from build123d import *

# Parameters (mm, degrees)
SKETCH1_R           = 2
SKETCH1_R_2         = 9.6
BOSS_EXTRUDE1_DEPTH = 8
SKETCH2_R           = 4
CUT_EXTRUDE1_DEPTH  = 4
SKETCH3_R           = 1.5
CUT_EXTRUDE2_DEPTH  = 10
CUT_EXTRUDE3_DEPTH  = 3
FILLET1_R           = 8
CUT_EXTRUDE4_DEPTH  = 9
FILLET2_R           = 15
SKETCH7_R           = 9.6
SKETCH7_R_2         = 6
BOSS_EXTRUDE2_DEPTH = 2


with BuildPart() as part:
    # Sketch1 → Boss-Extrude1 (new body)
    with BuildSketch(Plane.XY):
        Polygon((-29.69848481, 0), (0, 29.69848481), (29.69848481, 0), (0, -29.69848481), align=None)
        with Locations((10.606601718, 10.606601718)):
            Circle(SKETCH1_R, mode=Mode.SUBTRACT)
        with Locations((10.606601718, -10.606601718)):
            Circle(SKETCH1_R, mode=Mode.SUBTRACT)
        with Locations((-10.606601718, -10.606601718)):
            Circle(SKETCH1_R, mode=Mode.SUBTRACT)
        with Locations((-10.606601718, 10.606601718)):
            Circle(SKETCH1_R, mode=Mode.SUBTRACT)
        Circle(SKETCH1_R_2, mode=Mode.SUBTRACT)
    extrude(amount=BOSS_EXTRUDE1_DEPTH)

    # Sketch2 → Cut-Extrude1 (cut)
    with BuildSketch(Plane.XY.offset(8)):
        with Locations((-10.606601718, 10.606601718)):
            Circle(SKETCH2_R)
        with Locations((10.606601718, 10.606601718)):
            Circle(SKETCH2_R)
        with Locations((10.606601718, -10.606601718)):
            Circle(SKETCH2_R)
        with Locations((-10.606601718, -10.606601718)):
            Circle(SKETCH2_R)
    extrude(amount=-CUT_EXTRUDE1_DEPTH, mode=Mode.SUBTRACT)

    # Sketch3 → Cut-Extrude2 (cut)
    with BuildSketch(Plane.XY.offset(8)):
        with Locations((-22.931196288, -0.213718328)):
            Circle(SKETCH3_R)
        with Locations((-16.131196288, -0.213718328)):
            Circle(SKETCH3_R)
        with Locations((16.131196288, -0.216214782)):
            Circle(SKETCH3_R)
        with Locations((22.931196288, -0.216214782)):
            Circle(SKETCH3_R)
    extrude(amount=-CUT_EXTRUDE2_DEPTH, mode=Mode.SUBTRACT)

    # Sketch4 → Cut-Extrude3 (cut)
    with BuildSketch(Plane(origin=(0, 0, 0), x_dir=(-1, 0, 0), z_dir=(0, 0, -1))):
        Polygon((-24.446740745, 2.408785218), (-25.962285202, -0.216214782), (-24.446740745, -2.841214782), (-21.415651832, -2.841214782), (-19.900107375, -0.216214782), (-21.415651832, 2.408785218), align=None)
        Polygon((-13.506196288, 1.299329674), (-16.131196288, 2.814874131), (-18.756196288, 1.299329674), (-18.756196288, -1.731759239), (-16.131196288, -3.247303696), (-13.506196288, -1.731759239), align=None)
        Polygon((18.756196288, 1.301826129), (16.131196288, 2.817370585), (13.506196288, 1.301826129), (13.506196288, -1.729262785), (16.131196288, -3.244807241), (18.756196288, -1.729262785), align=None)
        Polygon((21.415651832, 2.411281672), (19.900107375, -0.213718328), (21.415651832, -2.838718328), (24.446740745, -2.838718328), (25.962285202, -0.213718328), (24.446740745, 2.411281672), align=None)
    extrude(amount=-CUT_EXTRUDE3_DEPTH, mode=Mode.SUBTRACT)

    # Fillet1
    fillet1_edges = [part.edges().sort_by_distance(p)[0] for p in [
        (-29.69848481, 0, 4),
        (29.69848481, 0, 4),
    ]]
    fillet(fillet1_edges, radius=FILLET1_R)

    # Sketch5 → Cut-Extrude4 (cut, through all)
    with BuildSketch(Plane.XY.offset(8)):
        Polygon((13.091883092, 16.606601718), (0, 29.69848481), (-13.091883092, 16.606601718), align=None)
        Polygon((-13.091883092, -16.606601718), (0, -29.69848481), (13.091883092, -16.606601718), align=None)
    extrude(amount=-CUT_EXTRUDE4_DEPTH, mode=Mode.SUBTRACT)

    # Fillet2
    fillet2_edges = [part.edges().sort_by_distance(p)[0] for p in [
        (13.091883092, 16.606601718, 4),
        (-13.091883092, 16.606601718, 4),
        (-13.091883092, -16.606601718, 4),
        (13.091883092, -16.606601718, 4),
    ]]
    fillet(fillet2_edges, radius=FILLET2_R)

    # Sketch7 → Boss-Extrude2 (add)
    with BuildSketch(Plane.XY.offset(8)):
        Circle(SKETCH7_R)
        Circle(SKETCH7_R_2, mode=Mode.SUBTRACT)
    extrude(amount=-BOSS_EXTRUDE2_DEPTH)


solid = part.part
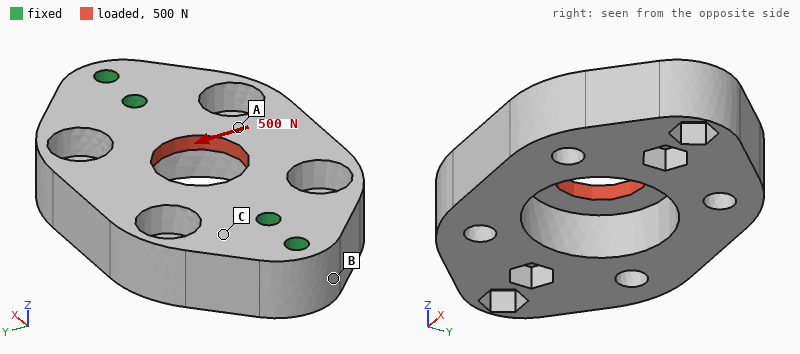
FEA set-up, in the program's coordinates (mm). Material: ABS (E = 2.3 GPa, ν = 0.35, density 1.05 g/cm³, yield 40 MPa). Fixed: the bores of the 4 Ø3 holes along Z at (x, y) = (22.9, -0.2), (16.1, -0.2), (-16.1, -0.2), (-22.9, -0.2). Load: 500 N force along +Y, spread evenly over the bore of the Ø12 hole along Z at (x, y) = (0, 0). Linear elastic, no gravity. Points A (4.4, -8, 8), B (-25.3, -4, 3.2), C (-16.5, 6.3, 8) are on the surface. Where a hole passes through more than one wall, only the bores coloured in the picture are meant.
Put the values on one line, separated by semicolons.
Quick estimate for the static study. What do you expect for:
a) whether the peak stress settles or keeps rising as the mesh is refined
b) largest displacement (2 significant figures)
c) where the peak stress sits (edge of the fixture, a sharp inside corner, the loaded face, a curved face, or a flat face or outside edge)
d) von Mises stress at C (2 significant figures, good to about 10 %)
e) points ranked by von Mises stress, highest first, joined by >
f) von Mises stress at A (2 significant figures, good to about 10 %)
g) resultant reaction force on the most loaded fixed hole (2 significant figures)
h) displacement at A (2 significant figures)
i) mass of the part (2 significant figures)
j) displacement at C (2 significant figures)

keeps rising; 0.10 mm; edge of the fixture; 4.1 MPa; A > C > B; 8.5 MPa; 250 N; 0.071 mm; 8.0 g; 0.016 mm
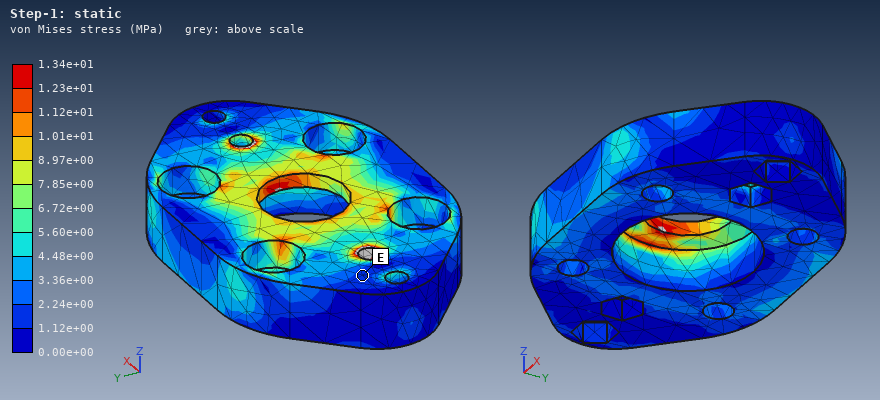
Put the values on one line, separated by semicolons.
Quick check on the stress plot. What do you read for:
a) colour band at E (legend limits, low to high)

1.12e+00 to 2.24e+00 MPa
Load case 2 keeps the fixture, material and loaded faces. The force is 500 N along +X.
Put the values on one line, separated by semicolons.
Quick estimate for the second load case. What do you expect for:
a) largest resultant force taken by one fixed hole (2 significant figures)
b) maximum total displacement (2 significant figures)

190 N; 47 µm
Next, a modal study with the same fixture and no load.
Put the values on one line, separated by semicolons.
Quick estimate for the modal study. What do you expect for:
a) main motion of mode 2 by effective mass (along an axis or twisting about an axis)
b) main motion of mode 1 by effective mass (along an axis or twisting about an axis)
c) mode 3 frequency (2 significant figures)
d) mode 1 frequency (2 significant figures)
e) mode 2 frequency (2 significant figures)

along Z; twisting about X; 7200 Hz; 3300 Hz; 4400 Hz
